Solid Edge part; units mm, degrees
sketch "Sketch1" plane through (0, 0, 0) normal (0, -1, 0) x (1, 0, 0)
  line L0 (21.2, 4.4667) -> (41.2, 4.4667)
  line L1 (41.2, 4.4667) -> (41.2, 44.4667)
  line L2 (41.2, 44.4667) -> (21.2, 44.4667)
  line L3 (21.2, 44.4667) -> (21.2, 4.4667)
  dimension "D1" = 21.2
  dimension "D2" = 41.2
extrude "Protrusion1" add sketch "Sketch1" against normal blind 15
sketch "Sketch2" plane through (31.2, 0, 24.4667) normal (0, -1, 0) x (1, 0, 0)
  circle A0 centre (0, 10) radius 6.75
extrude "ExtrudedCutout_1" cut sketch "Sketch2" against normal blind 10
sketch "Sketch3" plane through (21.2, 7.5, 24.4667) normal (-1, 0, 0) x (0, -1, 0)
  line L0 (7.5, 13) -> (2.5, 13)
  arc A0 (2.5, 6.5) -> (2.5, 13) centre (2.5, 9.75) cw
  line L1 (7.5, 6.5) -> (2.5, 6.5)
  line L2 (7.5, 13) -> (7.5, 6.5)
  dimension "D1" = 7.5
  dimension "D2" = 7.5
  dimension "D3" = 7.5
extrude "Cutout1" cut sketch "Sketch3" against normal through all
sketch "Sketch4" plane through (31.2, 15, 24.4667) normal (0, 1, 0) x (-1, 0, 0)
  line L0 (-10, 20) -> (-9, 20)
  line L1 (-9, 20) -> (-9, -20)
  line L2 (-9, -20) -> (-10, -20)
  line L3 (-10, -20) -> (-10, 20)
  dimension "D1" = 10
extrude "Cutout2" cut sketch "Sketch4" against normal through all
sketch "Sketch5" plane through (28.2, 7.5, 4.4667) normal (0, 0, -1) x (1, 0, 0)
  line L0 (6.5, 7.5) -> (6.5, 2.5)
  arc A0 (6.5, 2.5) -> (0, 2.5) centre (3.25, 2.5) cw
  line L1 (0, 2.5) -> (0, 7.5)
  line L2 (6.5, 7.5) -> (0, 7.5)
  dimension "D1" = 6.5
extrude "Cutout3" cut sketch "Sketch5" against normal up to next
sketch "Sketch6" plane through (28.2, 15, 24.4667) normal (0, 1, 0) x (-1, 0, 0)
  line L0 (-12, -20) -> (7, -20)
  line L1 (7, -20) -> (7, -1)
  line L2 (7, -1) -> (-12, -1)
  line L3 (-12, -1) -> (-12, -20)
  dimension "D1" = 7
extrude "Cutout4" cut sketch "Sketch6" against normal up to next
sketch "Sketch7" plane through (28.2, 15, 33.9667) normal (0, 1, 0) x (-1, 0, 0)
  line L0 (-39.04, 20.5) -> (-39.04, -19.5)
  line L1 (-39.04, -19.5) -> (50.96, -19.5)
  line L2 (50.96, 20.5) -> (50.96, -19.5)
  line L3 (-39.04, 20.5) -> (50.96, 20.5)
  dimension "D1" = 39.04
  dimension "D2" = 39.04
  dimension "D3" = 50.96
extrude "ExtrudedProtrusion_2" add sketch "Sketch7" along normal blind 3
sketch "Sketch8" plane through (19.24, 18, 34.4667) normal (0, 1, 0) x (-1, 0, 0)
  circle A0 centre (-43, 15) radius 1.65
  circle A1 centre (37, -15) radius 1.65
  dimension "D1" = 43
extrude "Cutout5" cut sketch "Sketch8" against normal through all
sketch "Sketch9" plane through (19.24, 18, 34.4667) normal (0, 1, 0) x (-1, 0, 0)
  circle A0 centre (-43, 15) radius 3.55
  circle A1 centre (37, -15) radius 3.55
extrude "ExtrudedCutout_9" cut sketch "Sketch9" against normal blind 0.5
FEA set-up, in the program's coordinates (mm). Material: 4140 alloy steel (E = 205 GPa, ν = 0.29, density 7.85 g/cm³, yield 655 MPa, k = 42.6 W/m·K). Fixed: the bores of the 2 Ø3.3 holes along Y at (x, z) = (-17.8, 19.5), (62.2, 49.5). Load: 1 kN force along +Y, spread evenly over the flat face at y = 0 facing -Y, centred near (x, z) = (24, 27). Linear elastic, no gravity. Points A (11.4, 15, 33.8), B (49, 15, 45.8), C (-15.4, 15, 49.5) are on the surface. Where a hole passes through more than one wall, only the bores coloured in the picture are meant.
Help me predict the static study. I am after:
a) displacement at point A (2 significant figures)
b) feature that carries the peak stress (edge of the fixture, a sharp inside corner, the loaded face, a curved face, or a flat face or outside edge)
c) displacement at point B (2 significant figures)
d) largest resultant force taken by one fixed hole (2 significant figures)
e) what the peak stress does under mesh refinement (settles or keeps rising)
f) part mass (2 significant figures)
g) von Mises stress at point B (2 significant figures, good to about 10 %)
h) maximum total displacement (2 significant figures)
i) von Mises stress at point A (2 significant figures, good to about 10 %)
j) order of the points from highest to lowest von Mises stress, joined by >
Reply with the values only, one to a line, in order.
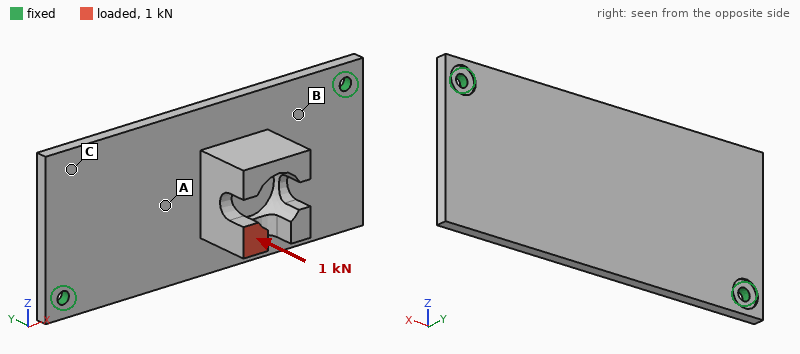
0.18 mm
edge of the fixture
0.060 mm
520 N
keeps rising
120 g
76 MPa
0.35 mm
140 MPa
A > B > C
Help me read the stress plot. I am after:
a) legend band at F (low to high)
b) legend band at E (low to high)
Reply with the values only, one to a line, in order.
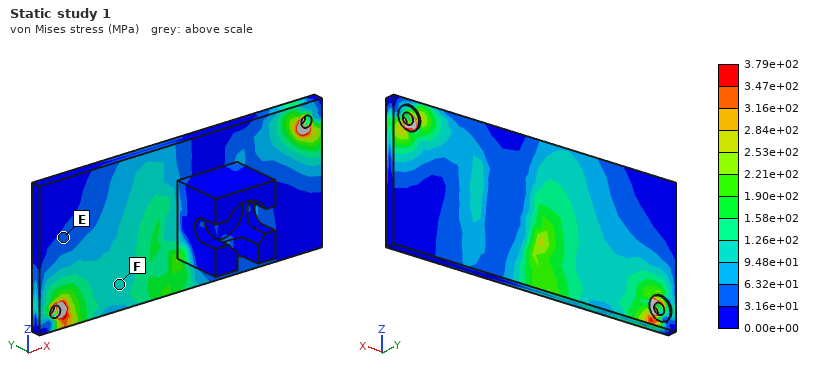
9.48e+01 to 1.26e+02 MPa
3.16e+01 to 6.32e+01 MPa
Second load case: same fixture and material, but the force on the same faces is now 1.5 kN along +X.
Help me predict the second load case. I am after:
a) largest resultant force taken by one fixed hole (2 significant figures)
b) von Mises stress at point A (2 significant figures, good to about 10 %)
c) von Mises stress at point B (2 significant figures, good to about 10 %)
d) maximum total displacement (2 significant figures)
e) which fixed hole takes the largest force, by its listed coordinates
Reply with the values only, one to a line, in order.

1.0 kN
110 MPa
120 MPa
0.23 mm
(62.2, 49.5)
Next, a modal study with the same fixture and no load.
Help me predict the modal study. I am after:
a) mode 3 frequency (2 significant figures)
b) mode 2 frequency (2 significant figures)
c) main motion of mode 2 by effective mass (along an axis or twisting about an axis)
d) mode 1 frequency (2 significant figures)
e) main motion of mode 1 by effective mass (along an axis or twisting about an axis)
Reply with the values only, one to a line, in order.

3400 Hz
1400 Hz
along Y
1300 Hz
along Y
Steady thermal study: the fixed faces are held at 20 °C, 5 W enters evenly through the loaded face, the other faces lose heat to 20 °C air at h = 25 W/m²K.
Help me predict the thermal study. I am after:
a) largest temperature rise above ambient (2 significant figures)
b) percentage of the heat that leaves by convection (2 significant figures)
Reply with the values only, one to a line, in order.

45 K
51 %
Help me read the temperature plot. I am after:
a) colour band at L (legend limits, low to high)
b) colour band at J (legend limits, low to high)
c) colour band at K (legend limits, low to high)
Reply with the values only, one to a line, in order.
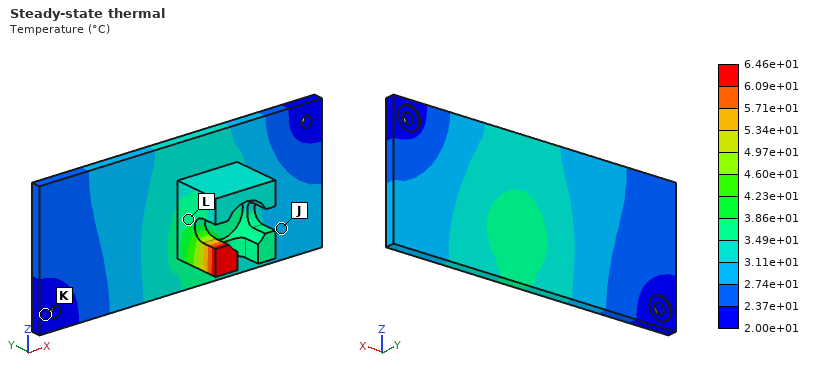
3.49e+01 to 3.86e+01 °C
2.74e+01 to 3.11e+01 °C
2.00e+01 to 2.37e+01 °C
